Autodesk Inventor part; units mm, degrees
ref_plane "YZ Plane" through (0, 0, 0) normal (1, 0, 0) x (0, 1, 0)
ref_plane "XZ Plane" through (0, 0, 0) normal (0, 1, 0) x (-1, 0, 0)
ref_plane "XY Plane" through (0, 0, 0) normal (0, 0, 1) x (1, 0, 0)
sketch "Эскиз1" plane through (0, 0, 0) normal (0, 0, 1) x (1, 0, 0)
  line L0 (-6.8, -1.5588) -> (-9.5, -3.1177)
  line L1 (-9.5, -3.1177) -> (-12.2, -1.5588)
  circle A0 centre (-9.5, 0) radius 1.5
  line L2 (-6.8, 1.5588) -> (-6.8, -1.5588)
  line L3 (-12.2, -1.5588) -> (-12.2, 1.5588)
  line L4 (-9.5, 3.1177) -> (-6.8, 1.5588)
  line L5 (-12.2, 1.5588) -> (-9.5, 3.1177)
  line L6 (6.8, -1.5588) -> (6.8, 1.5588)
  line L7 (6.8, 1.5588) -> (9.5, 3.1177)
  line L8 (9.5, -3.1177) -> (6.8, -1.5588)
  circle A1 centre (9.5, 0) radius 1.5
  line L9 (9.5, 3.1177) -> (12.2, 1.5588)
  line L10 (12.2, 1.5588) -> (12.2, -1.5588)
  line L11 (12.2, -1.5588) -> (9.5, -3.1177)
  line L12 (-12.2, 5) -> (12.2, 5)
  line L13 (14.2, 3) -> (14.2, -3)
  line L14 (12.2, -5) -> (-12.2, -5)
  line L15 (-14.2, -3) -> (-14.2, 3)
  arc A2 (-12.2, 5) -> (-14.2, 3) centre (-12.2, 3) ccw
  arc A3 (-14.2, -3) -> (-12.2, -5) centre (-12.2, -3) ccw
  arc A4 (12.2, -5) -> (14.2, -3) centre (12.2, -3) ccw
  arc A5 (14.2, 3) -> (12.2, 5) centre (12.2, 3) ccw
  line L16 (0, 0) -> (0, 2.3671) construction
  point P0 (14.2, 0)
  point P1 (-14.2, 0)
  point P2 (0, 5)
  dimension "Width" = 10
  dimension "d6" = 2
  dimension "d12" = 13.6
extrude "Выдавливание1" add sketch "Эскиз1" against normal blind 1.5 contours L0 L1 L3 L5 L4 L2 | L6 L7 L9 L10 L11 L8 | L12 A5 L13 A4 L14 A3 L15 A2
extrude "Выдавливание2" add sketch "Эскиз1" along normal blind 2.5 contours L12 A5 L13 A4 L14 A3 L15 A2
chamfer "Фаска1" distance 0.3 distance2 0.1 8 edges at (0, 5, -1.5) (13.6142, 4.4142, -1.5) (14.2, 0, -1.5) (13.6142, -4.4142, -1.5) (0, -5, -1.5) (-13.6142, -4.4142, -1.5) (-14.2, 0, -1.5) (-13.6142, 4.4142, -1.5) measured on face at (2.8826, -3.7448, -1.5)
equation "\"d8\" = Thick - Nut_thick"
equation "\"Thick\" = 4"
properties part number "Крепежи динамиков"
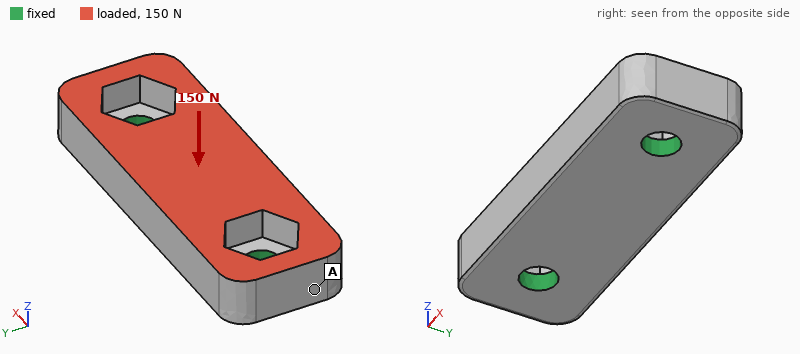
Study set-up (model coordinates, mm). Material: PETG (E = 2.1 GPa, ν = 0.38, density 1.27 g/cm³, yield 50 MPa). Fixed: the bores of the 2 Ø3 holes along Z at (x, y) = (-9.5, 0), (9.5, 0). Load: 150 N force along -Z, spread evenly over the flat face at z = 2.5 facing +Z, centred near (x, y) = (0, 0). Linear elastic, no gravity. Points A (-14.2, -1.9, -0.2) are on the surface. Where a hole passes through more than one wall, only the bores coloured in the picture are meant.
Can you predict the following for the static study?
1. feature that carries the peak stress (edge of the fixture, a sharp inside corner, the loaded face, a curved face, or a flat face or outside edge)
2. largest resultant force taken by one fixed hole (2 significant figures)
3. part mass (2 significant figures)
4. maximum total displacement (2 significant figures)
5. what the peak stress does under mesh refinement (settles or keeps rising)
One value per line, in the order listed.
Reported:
edge of the fixture
82 N
1.2 g
53 µm
keeps rising
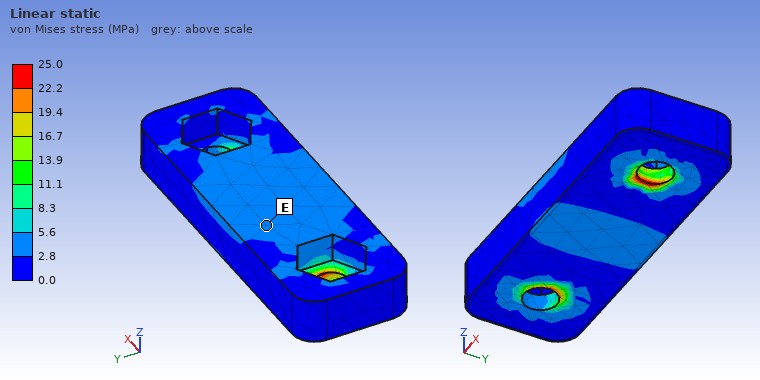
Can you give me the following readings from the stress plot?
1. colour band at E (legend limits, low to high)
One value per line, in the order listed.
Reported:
2.8 to 5.6 MPa
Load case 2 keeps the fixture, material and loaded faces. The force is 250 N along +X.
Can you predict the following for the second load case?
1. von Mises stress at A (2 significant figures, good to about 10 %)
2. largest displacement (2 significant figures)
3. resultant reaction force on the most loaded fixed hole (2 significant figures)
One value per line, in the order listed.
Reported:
1.9 MPa
56 µm
130 N
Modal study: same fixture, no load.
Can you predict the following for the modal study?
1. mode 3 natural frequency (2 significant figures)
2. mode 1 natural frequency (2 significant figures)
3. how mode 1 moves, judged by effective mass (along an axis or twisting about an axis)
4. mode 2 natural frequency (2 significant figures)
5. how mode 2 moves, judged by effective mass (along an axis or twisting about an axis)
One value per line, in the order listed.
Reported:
12 kHz
6800 Hz
along Y
8600 Hz
along Z
